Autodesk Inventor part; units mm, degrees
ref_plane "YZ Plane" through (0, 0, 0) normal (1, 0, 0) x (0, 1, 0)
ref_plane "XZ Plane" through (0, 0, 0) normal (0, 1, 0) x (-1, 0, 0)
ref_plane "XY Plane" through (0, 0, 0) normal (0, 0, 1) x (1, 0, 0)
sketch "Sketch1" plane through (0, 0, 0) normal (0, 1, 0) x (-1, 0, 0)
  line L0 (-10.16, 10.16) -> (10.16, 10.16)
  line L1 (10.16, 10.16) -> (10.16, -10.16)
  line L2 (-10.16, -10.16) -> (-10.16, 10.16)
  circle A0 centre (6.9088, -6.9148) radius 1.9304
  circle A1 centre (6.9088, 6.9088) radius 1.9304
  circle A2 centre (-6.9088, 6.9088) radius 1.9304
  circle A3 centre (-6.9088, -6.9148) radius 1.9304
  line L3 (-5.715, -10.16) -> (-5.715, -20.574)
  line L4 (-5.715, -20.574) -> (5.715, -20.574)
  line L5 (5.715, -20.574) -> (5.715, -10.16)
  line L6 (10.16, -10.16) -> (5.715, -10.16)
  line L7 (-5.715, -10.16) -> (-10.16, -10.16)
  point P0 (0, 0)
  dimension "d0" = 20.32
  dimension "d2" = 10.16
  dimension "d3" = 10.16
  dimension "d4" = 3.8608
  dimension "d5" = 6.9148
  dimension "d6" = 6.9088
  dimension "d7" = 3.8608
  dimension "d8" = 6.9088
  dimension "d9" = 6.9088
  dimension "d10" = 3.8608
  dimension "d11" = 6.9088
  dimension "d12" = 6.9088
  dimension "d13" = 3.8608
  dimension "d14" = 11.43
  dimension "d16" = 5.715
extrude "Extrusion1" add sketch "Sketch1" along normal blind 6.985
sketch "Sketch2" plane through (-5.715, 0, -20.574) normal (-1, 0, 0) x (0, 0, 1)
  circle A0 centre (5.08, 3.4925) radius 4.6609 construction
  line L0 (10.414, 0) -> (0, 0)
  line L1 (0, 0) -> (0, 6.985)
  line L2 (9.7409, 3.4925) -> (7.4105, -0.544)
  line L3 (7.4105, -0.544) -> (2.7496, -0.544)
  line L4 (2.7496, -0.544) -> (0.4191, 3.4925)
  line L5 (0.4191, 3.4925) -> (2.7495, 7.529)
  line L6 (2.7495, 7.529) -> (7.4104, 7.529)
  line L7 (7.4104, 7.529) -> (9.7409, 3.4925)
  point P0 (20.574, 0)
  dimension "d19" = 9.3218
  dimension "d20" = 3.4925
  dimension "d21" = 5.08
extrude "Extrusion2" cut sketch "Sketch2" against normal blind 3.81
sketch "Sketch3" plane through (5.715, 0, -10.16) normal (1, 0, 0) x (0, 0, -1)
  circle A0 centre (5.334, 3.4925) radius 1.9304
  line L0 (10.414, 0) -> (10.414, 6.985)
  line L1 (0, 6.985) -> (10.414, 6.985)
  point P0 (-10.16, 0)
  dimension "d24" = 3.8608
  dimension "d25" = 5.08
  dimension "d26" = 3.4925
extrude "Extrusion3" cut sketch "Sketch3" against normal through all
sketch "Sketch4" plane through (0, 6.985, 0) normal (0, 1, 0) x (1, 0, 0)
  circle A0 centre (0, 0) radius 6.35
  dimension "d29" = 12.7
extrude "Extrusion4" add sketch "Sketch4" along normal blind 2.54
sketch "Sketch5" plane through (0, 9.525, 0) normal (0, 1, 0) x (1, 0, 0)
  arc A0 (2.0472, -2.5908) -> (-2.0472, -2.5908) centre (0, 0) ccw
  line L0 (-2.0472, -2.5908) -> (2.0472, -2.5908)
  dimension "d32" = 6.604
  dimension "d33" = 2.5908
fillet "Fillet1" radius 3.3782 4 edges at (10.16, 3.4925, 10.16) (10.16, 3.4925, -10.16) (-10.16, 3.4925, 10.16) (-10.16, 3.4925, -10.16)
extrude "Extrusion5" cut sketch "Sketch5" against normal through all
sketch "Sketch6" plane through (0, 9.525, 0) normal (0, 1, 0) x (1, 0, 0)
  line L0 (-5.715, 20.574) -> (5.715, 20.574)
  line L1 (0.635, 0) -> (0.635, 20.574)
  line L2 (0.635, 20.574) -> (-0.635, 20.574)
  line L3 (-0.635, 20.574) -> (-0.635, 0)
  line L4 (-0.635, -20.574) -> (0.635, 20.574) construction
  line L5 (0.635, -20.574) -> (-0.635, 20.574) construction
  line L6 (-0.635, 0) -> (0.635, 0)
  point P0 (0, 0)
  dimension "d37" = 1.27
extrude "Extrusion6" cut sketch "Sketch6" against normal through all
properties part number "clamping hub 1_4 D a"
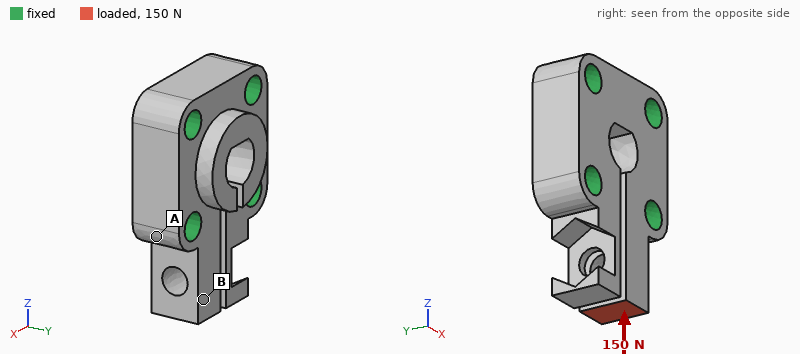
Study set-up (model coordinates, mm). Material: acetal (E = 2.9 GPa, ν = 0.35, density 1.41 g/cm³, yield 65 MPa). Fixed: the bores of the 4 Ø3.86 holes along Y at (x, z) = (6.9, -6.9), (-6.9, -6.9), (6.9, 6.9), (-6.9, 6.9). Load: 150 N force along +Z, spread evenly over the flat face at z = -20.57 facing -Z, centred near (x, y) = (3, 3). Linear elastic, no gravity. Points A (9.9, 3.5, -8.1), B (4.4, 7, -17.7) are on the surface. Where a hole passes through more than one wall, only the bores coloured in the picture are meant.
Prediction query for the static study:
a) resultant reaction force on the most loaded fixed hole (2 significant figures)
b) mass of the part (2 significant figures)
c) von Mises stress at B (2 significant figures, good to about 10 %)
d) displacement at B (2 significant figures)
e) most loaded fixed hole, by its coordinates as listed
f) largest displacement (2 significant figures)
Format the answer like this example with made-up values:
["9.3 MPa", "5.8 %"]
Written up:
["130 N", "4.1 g", "6.8 MPa", "33 µm", "(6.9, -6.9)", "57 µm"]
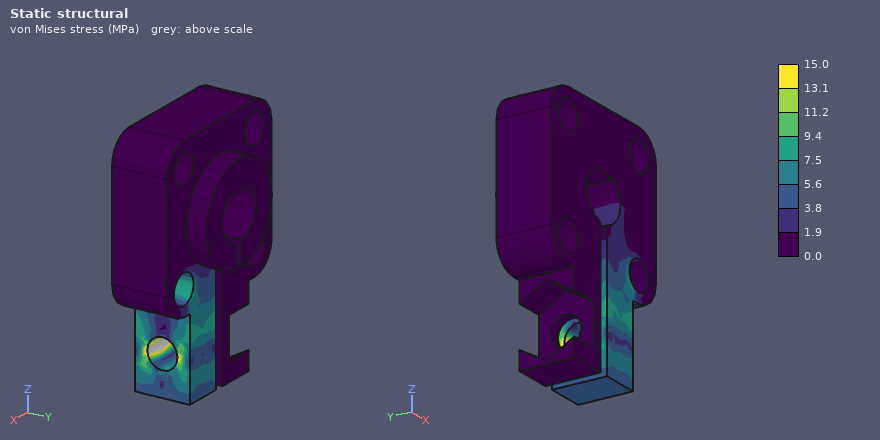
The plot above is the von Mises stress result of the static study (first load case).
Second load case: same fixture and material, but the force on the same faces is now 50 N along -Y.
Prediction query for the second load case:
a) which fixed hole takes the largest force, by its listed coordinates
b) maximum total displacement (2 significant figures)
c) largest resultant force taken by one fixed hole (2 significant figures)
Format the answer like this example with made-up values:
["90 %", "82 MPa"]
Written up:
["(6.9, -6.9)", "0.16 mm", "59 N"]
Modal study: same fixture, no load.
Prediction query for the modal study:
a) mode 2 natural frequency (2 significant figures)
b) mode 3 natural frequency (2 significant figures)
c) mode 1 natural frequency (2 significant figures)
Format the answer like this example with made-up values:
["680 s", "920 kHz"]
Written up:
["3800 Hz", "6300 Hz", "1800 Hz"]
